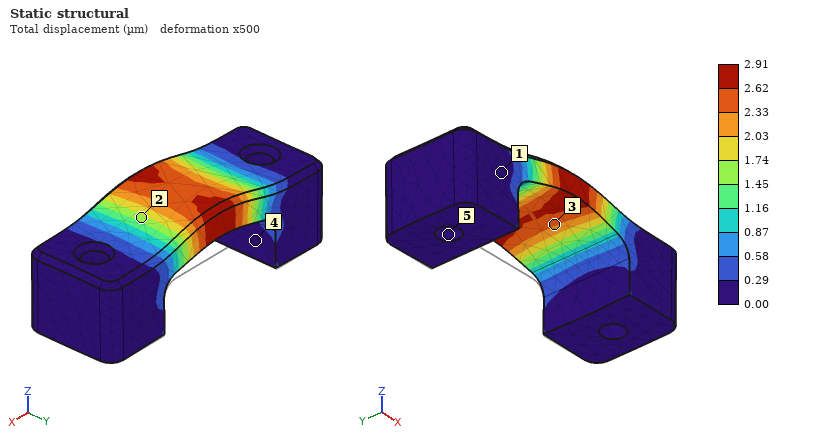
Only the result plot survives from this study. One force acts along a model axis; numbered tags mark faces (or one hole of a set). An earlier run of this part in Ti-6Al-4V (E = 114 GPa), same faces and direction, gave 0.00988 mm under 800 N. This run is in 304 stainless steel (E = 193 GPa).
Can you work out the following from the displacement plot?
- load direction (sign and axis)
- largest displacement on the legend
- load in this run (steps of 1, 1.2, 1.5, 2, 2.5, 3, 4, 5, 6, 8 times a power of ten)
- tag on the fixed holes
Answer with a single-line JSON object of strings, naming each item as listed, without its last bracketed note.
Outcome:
{"load direction": "+Z", "largest displacement on the legend": "2.91 µm", "load in this run": "400 N", "tag on the fixed holes": "5"}
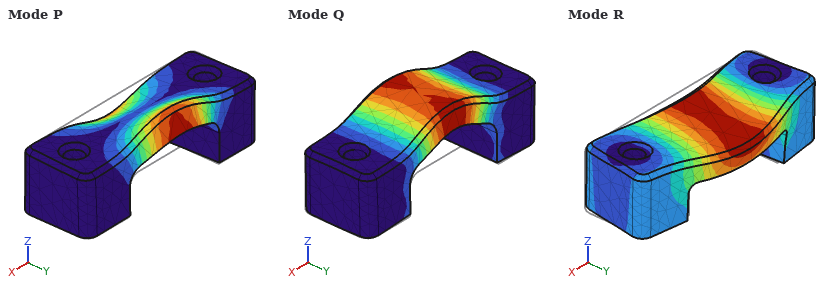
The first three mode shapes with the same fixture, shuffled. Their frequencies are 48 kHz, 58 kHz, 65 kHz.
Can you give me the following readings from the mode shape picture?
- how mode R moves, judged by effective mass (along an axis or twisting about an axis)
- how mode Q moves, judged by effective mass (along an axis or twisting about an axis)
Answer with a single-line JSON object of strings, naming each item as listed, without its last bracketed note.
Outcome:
{"how mode R moves, judged by effective mass": "along Y", "how mode Q moves, judged by effective mass": "along Z"}
